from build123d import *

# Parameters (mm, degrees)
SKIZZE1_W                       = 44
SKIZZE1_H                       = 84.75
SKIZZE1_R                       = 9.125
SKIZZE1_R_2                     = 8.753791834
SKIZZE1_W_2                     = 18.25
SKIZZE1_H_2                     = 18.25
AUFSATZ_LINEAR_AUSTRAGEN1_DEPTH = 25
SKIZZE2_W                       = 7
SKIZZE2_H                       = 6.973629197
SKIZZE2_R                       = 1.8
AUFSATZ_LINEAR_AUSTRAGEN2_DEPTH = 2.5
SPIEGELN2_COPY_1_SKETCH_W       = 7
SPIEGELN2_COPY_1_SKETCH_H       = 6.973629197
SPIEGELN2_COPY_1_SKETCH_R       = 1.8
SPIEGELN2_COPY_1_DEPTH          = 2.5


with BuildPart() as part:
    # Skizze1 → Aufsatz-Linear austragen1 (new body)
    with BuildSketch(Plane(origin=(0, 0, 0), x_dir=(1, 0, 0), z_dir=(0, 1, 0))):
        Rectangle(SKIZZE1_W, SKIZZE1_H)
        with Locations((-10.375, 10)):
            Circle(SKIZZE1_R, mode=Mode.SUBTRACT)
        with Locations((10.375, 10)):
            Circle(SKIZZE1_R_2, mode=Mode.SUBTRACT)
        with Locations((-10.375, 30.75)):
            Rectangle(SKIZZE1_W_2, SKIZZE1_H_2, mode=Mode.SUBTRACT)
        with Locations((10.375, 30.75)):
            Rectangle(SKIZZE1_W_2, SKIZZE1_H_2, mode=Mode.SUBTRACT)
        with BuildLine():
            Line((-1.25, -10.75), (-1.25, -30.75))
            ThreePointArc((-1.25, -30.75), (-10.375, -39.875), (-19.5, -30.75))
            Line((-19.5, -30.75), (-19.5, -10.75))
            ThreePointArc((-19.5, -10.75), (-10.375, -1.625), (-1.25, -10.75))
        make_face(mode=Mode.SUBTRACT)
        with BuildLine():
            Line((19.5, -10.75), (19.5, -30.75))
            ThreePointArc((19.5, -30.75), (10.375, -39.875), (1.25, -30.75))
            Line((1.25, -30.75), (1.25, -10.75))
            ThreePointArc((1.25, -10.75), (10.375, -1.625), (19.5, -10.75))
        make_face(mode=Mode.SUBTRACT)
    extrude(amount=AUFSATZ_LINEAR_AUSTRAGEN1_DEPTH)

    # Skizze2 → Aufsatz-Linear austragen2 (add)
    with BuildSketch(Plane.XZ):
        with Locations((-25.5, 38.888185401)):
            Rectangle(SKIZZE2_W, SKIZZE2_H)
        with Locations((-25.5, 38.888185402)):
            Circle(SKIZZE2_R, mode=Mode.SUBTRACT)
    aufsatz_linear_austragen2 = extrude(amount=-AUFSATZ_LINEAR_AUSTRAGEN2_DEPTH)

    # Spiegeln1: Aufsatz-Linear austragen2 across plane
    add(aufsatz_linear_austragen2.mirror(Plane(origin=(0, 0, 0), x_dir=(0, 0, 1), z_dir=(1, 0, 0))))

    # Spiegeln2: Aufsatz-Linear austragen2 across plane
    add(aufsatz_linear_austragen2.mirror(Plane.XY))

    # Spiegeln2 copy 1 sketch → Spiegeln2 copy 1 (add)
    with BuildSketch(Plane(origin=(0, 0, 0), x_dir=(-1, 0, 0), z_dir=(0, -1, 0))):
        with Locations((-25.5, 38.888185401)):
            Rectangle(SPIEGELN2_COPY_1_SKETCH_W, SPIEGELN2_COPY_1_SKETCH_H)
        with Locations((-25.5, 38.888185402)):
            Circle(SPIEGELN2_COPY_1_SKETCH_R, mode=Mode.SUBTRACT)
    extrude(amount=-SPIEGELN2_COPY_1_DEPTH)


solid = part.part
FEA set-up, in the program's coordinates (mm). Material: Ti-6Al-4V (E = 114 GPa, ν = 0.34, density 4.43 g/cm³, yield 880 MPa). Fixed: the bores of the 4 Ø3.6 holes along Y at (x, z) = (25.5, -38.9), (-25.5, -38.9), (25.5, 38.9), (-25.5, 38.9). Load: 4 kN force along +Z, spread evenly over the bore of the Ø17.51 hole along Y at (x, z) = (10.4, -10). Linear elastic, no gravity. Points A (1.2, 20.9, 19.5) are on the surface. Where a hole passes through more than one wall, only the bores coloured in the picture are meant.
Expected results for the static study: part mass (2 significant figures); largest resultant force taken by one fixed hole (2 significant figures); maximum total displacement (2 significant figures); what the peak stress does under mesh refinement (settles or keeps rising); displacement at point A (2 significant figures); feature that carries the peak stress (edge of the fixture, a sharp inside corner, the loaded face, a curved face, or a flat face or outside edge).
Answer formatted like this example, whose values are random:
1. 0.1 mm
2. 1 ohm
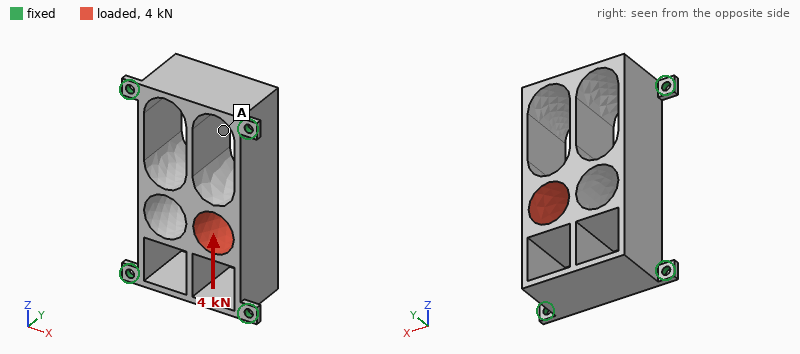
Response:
1. 150 g
2. 1.5 kN
3. 32 µm
4. keeps rising
5. 28 µm
6. edge of the fixture
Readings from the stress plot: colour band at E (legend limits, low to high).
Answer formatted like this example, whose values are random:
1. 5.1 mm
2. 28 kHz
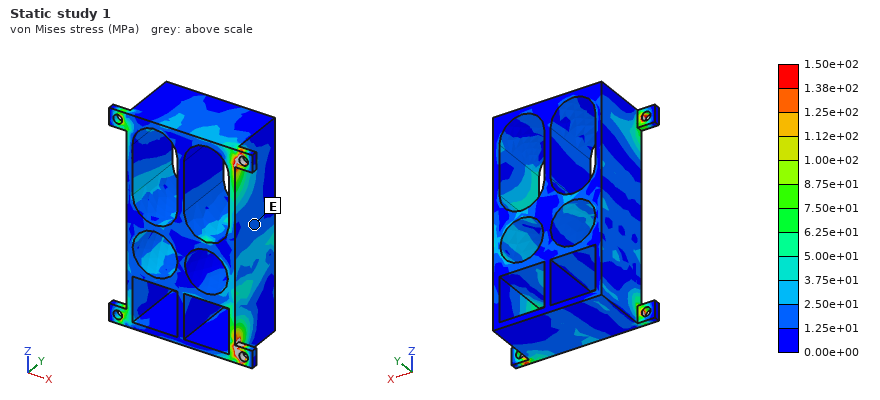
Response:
1. 1.25e+01 to 2.50e+01 MPa
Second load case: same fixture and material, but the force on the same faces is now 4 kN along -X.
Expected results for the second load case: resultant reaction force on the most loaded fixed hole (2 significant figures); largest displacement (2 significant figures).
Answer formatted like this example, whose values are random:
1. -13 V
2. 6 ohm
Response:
1. 1.7 kN
2. 0.21 mm
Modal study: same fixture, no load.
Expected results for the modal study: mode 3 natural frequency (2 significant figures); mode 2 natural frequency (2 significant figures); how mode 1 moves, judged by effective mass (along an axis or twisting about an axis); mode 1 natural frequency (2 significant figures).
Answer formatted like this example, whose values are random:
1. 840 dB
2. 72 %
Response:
1. 5600 Hz
2. 5500 Hz
3. along X
4. 2500 Hz
